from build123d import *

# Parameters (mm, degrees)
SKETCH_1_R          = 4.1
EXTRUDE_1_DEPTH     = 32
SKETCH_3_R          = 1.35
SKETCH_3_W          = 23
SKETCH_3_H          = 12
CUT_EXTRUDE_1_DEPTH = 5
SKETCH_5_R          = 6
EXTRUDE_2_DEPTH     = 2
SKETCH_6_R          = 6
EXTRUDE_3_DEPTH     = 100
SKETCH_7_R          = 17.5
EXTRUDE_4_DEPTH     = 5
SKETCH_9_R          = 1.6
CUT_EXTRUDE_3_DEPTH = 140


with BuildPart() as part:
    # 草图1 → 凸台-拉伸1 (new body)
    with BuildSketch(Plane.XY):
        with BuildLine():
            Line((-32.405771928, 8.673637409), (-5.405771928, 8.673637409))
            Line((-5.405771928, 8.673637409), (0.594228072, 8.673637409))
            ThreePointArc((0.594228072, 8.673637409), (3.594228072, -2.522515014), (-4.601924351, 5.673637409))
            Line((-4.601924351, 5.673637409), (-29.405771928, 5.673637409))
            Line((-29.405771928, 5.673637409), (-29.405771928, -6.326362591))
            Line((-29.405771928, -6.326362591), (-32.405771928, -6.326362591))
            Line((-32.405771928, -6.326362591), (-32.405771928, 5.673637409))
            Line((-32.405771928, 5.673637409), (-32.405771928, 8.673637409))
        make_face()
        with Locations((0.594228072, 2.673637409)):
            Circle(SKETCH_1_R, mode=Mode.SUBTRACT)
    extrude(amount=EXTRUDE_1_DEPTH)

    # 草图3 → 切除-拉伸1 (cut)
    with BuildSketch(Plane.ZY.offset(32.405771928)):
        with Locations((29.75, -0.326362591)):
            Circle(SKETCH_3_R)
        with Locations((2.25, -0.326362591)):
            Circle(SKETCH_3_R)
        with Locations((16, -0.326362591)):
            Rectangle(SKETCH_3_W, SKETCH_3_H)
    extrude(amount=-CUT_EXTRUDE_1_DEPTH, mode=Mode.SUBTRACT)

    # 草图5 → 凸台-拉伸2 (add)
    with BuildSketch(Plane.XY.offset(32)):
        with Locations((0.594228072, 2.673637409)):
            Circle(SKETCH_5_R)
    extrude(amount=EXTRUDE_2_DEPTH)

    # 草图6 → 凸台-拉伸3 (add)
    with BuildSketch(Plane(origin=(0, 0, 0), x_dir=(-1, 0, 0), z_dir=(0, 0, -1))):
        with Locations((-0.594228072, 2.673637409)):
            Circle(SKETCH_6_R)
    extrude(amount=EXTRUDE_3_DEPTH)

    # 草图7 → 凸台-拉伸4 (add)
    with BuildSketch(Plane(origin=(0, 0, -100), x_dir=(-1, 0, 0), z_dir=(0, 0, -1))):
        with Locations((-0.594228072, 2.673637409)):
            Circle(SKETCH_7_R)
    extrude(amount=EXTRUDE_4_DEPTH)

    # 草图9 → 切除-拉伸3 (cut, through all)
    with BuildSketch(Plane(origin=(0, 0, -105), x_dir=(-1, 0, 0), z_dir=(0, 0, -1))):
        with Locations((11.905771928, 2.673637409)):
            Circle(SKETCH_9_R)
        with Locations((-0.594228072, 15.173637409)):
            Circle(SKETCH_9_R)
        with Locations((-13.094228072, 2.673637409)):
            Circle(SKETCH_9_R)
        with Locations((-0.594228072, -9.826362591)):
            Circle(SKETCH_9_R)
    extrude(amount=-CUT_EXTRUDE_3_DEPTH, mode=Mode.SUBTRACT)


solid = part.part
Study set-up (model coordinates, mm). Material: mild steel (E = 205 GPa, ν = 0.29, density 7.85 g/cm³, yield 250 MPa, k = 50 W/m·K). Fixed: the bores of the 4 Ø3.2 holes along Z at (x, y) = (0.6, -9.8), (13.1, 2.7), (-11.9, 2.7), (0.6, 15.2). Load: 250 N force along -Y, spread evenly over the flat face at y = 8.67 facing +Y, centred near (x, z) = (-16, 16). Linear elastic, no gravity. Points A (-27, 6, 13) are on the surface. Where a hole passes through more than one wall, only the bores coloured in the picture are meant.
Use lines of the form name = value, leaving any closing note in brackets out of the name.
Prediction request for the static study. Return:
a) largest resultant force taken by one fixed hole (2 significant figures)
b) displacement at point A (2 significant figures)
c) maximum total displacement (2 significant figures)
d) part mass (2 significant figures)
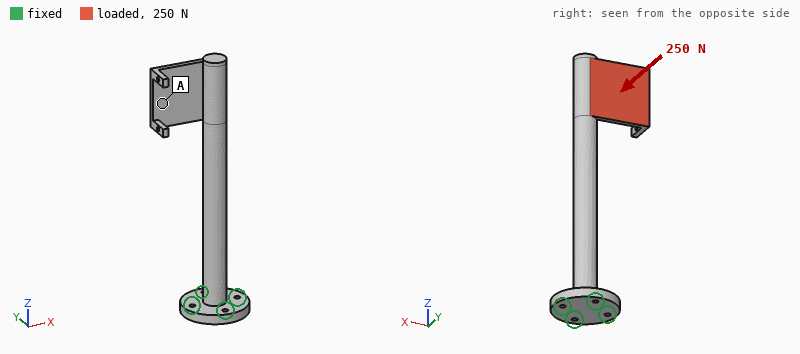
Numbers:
largest resultant force taken by one fixed hole = 1.3 kN
displacement at point A = 0.81 mm
maximum total displacement = 1.0 mm
part mass = 170 g
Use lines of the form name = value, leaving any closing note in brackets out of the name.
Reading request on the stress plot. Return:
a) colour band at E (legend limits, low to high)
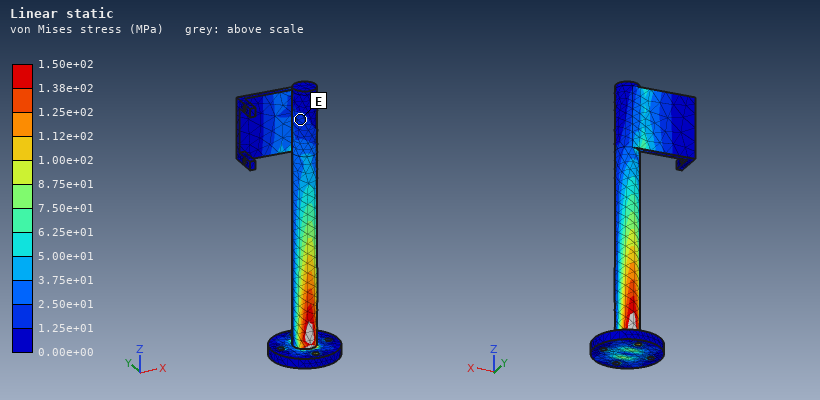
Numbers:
colour band at E = 1.25e+01 to 2.50e+01 MPa
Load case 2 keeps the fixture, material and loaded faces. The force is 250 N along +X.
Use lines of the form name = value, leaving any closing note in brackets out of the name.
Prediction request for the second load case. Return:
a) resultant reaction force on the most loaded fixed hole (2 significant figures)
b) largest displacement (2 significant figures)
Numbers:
resultant reaction force on the most loaded fixed hole = 1.3 kN
largest displacement = 0.91 mm
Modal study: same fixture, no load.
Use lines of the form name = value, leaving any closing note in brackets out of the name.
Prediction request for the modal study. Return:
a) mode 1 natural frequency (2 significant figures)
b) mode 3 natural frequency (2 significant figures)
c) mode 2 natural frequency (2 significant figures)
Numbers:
mode 1 natural frequency = 390 Hz
mode 3 natural frequency = 1600 Hz
mode 2 natural frequency = 390 Hz
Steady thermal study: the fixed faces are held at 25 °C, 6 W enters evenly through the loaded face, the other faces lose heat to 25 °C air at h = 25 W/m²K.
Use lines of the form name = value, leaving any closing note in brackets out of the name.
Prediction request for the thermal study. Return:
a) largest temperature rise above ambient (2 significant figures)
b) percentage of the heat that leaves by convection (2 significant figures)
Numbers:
largest temperature rise above ambient = 47 K
percentage of the heat that leaves by convection = 81 %
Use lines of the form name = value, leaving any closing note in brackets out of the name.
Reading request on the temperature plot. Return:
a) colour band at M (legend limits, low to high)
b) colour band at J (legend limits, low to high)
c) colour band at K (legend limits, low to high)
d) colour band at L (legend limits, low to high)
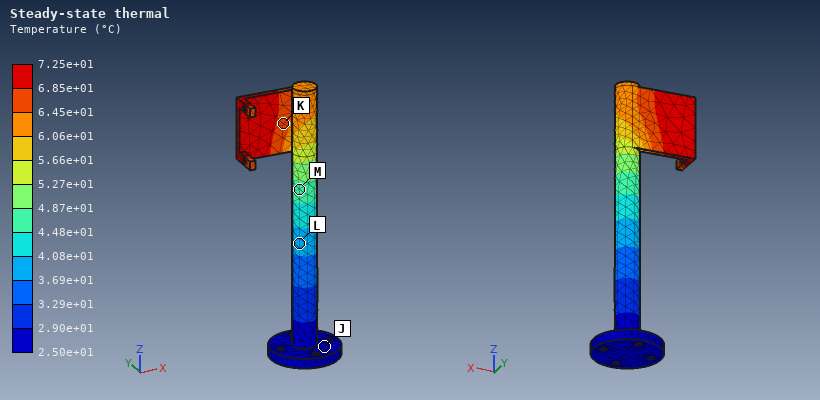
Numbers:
colour band at M = 4.48e+01 to 4.87e+01 °C
colour band at J = 2.50e+01 to 2.90e+01 °C
colour band at K = 6.45e+01 to 6.85e+01 °C
colour band at L = 3.69e+01 to 4.08e+01 °C
